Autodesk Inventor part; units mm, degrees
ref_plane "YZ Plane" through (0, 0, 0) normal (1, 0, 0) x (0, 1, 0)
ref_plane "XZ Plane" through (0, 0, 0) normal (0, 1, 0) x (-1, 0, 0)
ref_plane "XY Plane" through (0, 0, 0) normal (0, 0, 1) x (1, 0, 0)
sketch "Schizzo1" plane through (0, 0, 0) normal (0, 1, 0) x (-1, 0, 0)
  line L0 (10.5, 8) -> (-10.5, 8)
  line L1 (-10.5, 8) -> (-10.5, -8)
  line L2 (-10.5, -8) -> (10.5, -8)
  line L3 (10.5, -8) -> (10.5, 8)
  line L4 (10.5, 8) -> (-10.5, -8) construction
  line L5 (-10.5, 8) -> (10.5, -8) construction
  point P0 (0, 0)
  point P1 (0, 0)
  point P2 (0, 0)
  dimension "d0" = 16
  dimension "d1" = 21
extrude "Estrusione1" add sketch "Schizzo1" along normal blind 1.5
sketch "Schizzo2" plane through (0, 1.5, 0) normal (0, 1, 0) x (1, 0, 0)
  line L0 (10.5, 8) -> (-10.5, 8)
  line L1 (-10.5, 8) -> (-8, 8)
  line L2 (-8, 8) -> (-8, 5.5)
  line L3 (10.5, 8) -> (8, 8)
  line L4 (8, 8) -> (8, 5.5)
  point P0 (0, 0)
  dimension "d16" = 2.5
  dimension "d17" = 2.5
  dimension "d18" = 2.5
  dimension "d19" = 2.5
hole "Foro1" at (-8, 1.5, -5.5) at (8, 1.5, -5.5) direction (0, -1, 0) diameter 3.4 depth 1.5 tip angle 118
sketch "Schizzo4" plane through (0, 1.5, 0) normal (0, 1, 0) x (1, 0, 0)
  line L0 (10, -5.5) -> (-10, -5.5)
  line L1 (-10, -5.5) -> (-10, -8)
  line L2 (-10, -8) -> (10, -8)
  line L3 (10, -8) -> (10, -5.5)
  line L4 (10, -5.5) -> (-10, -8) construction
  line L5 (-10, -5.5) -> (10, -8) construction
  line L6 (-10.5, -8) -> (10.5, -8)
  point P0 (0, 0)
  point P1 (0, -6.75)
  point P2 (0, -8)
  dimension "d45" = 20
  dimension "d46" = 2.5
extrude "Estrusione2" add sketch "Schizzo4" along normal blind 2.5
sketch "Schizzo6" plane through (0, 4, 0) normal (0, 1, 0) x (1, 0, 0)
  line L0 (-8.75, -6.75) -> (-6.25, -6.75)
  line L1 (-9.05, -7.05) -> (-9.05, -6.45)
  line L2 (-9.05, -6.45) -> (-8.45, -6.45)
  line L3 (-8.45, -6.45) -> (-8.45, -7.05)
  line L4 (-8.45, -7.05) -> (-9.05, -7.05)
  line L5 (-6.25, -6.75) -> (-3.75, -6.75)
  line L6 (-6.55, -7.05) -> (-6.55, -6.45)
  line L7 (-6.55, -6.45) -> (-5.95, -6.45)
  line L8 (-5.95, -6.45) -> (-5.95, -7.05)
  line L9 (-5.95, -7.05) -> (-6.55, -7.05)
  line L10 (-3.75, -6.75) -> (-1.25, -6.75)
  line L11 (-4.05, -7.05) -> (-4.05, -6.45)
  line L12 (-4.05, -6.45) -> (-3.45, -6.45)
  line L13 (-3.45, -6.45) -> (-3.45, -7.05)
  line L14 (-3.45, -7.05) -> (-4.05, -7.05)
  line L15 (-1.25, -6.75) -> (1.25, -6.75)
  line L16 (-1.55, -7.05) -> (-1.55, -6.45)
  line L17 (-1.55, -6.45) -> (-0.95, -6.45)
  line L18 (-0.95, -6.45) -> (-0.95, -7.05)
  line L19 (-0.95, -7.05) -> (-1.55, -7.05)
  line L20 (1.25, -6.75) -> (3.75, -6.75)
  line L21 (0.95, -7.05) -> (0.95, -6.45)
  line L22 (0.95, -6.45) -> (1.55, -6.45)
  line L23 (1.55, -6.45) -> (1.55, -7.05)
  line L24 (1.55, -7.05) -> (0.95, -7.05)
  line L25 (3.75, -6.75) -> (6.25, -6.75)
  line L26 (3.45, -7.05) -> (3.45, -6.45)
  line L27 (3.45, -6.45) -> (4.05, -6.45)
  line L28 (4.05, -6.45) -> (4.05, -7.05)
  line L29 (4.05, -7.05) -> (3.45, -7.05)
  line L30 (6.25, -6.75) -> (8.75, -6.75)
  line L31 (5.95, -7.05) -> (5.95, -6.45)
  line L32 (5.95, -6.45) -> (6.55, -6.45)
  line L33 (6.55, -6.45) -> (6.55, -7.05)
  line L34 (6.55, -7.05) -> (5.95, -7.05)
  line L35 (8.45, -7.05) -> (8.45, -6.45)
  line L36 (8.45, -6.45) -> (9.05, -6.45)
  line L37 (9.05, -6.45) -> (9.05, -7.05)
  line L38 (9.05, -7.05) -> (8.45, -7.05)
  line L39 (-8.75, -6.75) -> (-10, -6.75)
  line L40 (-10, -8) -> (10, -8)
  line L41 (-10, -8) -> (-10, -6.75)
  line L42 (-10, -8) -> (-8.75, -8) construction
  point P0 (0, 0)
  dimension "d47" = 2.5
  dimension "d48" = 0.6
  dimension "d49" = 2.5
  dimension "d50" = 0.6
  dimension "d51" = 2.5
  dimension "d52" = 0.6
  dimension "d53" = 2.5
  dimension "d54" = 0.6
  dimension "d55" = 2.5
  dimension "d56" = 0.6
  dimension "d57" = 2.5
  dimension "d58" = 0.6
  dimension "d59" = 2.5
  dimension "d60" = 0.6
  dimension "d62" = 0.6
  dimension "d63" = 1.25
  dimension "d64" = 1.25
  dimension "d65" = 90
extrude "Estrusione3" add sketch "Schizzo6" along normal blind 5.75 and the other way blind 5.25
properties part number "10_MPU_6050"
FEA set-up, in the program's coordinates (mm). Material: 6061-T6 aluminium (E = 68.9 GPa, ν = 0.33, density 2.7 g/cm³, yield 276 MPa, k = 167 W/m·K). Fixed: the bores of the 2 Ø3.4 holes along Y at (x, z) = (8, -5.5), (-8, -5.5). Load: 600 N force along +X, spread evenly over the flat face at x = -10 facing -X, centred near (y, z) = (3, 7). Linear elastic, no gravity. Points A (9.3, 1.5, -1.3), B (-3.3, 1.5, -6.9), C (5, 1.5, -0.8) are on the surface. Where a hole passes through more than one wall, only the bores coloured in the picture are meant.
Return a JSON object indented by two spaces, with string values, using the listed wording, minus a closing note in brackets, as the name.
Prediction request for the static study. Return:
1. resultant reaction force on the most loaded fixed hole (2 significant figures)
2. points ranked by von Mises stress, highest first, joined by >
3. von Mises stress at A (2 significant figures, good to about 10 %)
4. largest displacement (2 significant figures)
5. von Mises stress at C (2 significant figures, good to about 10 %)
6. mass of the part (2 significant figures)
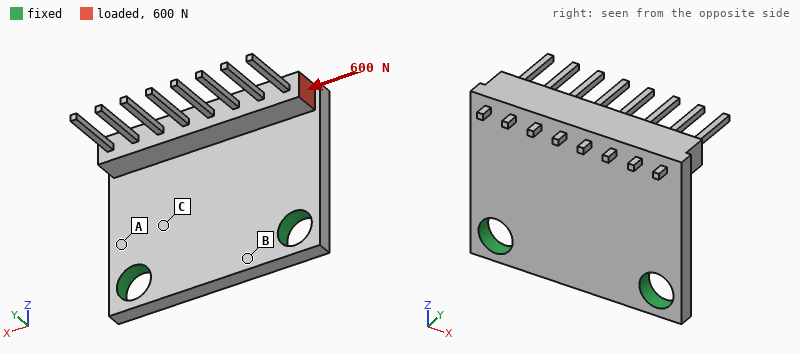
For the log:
{
  "resultant reaction force on the most loaded fixed hole": "520 N",
  "points ranked by von Mises stress, highest first, joined by >": "C > A > B",
  "von Mises stress at A": "59 MPa",
  "largest displacement": "0.13 mm",
  "von Mises stress at C": "91 MPa",
  "mass of the part": "1.7 g"
}
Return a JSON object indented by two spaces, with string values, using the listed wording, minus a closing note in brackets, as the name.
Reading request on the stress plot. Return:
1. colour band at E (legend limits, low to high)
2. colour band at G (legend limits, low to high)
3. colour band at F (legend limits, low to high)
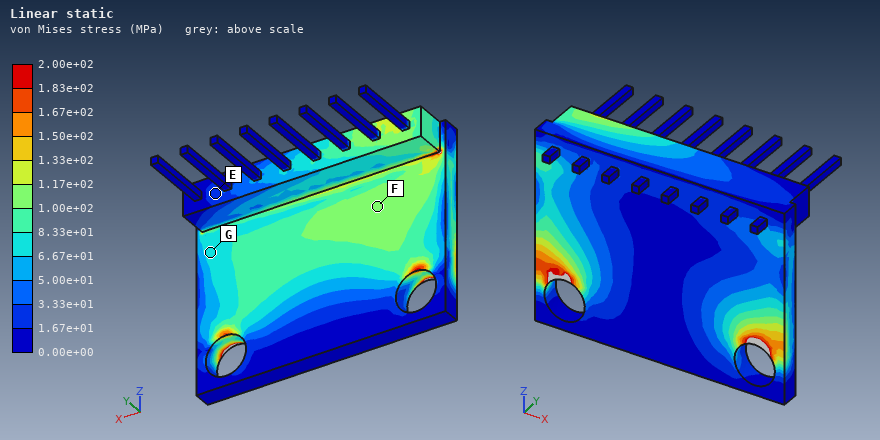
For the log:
{
  "colour band at E": "1.67e+01 to 3.33e+01 MPa",
  "colour band at G": "6.67e+01 to 8.33e+01 MPa",
  "colour band at F": "1.00e+02 to 1.17e+02 MPa"
}
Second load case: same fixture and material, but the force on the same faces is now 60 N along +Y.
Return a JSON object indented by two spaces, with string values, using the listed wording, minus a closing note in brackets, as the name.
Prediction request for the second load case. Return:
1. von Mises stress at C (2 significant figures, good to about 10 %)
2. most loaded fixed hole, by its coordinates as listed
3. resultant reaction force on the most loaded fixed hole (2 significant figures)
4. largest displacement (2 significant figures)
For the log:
{
  "von Mises stress at C": "41 MPa",
  "most loaded fixed hole, by its coordinates as listed": "(-8, -5.5)",
  "resultant reaction force on the most loaded fixed hole": "67 N",
  "largest displacement": "0.16 mm"
}
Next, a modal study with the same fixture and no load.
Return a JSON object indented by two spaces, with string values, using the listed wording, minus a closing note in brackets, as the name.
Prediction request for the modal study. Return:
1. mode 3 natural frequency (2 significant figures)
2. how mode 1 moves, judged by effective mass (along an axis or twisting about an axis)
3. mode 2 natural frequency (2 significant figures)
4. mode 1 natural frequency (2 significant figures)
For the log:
{
  "mode 3 natural frequency": "14 kHz",
  "how mode 1 moves, judged by effective mass": "along Y",
  "mode 2 natural frequency": "11 kHz",
  "mode 1 natural frequency": "4900 Hz"
}
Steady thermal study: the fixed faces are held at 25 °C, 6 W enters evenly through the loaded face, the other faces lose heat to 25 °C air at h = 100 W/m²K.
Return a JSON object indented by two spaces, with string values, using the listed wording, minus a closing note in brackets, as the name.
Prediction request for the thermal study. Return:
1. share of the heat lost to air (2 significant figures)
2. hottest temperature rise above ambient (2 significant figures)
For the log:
{
  "share of the heat lost to air": "13 %",
  "hottest temperature rise above ambient": "32 K"
}
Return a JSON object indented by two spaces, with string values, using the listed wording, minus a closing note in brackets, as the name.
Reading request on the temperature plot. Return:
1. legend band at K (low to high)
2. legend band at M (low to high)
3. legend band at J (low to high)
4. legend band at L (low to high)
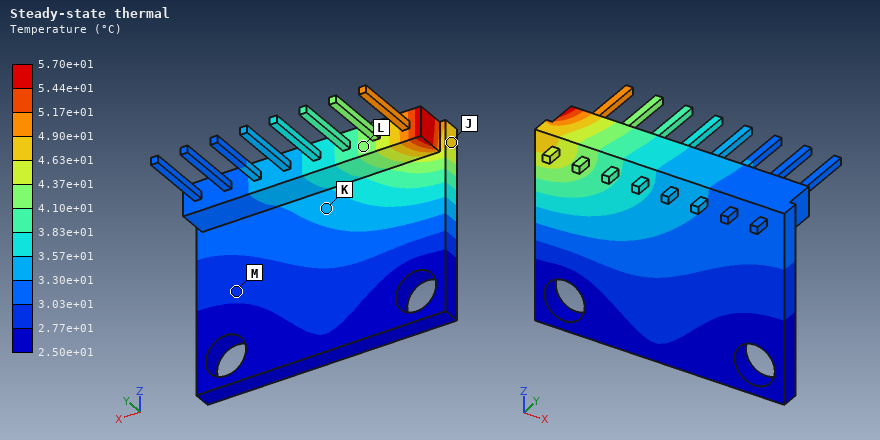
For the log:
{
  "legend band at K": "3.30e+01 to 3.57e+01 °C",
  "legend band at M": "2.77e+01 to 3.03e+01 °C",
  "legend band at J": "4.63e+01 to 4.90e+01 °C",
  "legend band at L": "4.10e+01 to 4.37e+01 °C"
}
